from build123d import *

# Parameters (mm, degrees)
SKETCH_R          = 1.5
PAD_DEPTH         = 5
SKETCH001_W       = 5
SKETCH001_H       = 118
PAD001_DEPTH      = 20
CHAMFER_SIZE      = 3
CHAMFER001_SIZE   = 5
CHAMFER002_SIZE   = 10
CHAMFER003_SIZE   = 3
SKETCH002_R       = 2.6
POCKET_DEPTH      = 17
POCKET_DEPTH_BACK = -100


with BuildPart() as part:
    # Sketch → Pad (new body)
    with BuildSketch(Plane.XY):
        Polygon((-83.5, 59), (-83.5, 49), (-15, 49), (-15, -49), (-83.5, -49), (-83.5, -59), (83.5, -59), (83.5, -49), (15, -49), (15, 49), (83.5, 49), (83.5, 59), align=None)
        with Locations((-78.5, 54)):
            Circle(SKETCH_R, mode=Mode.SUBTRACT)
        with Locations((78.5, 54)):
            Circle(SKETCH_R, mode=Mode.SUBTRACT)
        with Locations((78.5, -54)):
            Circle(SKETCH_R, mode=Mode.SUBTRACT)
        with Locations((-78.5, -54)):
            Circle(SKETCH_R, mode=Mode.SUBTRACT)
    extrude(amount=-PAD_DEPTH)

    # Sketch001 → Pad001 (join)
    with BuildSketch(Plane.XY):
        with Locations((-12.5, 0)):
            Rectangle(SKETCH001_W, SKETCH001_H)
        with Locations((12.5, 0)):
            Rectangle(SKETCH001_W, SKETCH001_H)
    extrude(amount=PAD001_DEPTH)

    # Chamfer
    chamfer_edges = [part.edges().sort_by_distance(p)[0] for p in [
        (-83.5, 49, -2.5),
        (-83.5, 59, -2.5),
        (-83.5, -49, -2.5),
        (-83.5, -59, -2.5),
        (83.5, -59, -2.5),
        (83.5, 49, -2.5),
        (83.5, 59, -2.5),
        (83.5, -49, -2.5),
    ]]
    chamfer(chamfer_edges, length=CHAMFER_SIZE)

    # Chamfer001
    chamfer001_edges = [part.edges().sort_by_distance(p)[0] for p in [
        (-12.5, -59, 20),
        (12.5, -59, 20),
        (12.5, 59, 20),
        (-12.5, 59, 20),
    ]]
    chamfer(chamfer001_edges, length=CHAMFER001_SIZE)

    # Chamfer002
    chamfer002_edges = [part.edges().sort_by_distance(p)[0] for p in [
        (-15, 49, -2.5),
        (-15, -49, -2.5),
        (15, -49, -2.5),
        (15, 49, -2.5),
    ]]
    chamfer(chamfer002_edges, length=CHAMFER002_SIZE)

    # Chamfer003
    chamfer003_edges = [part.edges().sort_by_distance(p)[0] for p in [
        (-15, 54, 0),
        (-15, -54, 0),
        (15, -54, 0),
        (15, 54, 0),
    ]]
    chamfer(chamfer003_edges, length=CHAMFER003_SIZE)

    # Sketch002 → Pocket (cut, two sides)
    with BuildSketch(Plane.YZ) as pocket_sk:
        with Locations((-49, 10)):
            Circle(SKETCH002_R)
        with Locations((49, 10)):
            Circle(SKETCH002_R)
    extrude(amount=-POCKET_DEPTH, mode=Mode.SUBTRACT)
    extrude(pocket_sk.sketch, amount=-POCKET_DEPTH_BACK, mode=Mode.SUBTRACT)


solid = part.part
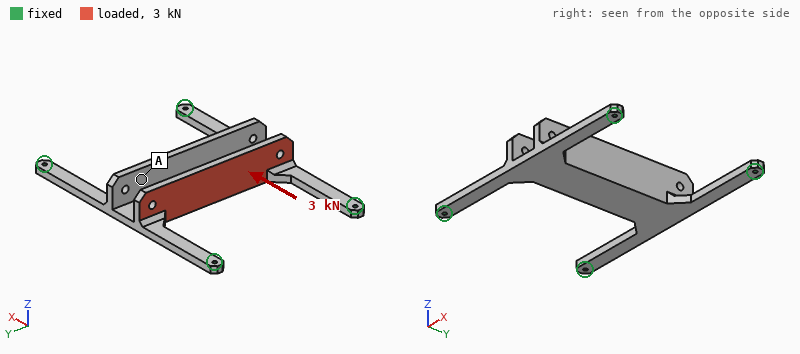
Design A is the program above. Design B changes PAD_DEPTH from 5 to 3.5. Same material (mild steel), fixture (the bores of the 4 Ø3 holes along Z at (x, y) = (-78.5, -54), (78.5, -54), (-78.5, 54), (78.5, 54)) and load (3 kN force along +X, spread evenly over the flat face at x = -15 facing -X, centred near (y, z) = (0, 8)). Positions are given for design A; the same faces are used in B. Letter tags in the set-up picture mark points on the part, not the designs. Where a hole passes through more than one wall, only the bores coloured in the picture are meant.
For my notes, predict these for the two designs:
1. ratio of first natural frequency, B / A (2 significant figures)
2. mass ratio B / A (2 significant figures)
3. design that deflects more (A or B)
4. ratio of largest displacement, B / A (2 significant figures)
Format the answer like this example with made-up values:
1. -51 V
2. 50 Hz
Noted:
1. 0.66
2. 0.83
3. B
4. 2.1
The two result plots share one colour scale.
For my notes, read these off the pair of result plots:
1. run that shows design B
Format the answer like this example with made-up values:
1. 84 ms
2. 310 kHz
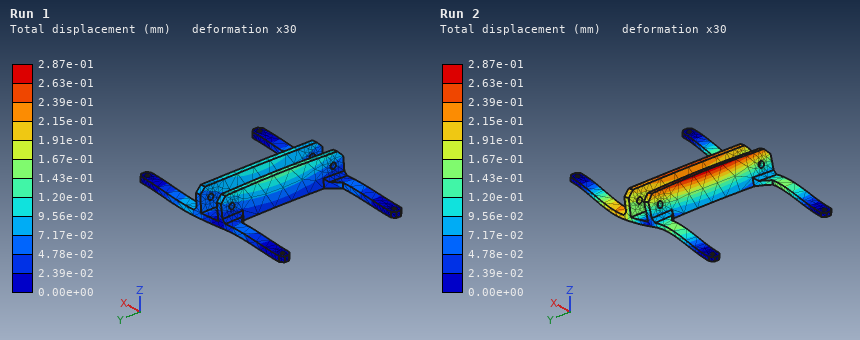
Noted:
1. Run 2
